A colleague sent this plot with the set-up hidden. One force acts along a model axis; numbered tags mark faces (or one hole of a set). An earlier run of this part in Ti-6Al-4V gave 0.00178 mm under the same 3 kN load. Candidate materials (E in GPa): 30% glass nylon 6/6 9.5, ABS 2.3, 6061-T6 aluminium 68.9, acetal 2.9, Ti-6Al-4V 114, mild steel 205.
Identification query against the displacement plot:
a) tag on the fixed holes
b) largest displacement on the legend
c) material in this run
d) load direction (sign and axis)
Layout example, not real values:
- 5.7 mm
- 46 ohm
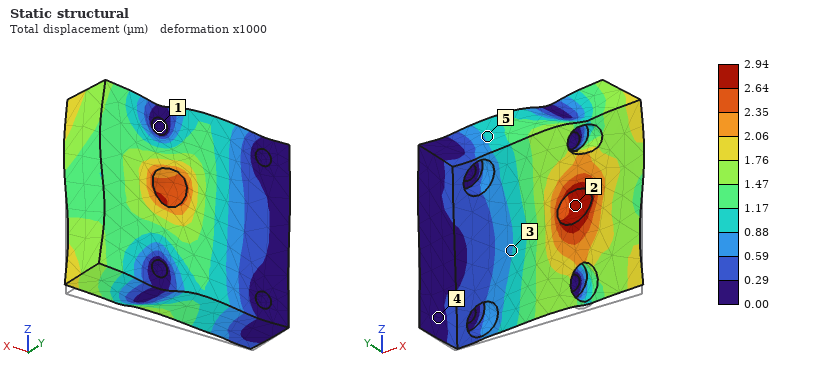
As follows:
- 1
- 2.94 µm
- 6061-T6 aluminium
- +Z
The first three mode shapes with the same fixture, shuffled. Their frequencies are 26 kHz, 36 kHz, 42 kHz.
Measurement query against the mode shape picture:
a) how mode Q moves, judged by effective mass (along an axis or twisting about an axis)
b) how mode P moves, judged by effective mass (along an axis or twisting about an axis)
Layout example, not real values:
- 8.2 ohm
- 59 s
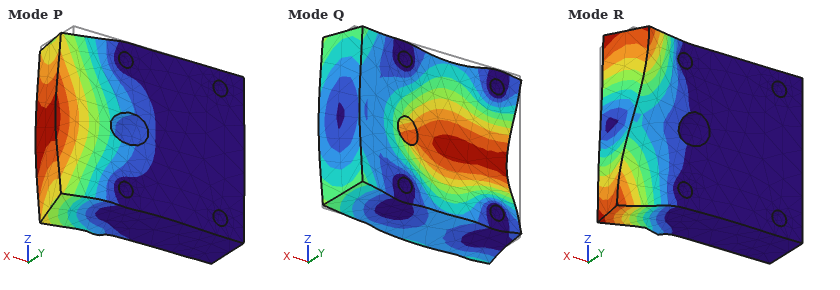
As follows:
- along Y
- along Y
